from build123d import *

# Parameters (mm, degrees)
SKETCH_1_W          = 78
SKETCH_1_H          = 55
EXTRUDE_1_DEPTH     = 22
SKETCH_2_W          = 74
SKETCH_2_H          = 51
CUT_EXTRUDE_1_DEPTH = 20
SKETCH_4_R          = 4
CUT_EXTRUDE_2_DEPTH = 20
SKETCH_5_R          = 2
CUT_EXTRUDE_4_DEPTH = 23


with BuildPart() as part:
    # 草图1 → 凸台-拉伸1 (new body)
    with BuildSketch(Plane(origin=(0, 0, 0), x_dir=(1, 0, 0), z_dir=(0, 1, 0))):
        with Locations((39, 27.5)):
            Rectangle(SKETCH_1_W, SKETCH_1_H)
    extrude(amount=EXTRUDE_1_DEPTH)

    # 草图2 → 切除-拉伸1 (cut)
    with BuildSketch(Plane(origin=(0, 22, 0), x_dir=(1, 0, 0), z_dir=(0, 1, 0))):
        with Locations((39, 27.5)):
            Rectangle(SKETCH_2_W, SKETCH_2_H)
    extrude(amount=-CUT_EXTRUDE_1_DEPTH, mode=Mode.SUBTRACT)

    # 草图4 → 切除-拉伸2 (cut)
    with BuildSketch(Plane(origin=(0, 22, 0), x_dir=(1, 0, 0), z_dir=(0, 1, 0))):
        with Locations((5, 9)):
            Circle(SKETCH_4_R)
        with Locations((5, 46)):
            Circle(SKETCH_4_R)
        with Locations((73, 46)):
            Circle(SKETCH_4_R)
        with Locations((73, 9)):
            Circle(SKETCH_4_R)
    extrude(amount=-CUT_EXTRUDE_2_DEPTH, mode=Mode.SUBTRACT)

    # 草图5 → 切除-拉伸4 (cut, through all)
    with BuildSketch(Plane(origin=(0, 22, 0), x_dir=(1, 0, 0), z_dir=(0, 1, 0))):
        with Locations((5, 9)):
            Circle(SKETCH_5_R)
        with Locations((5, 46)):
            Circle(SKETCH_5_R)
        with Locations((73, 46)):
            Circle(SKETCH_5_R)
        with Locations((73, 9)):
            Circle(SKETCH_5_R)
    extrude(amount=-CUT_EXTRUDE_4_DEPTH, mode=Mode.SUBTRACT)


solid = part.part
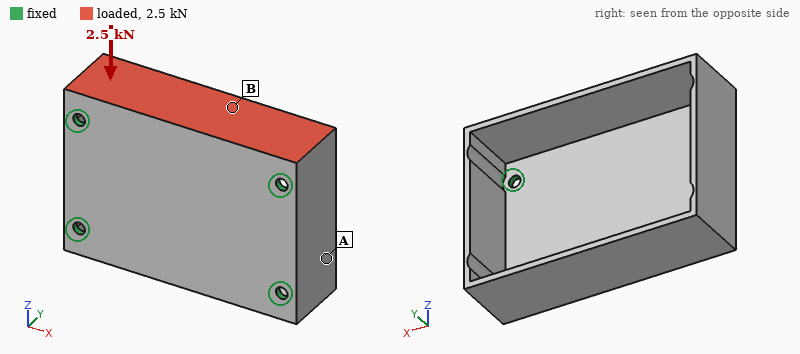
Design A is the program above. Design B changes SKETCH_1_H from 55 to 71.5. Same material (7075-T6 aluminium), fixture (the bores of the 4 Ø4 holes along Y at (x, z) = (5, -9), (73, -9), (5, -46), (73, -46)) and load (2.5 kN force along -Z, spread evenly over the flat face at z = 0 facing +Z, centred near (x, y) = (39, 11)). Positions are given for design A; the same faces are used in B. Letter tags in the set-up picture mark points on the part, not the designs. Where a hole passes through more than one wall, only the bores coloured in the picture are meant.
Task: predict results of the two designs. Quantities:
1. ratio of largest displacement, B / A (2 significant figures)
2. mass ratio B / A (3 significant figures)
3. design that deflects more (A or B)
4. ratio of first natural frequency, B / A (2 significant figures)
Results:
0.075
2.53
A
1.2
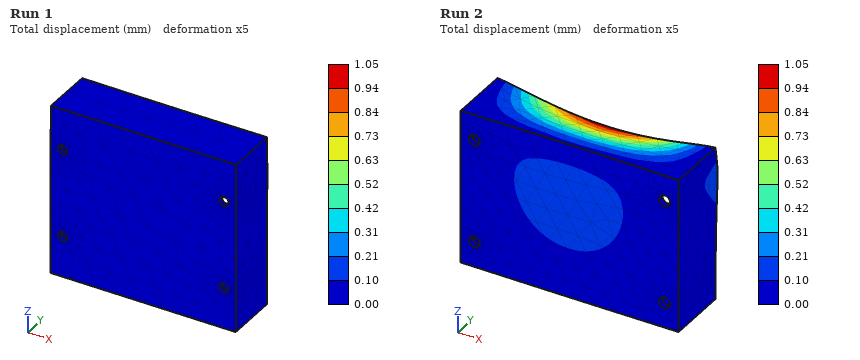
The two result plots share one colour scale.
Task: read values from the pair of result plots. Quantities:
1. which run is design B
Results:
Run 1
